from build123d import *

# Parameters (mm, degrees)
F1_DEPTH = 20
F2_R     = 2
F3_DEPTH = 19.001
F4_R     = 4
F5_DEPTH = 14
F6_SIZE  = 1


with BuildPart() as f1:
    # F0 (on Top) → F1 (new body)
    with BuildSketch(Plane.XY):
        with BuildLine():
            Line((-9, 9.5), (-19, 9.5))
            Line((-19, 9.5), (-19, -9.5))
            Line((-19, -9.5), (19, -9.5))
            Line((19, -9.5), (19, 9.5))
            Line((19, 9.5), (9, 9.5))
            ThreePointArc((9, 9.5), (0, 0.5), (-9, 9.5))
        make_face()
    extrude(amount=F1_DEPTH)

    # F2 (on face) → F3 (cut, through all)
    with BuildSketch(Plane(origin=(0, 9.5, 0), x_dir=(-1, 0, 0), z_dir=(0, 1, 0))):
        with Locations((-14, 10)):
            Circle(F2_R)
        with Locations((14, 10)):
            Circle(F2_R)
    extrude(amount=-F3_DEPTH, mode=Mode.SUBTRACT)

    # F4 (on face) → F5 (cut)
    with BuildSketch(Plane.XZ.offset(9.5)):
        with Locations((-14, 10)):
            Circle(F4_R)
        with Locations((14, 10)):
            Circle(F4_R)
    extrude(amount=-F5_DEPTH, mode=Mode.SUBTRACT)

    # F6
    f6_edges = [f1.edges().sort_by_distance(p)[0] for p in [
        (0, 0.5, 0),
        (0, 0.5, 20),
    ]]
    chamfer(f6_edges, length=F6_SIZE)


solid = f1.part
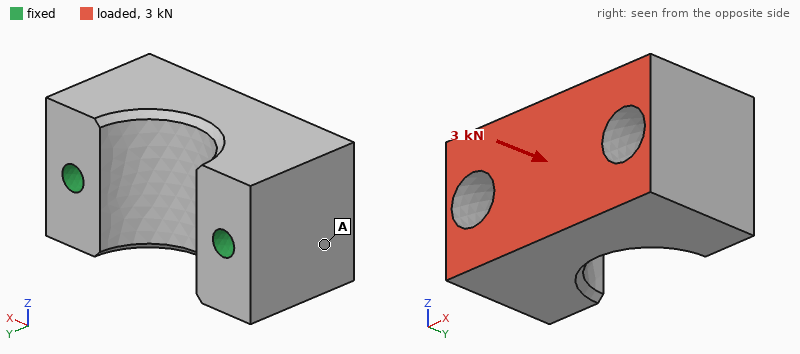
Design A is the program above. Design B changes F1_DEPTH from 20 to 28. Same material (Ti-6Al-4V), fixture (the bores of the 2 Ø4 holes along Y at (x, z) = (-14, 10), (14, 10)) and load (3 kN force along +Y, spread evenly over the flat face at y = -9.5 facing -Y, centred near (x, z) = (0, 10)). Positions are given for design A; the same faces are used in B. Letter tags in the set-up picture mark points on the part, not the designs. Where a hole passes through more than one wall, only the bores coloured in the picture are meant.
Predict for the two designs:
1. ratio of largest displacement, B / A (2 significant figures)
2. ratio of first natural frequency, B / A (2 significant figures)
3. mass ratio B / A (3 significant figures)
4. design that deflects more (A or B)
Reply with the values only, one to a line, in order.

6.1
0.71
1.46
B
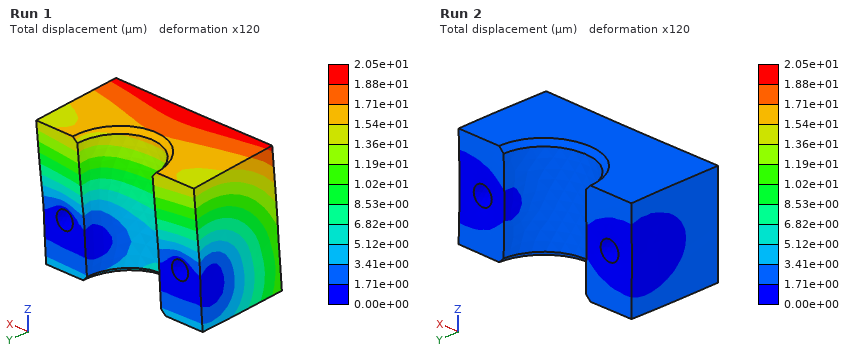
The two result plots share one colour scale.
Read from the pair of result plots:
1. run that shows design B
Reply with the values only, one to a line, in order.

Run 1
